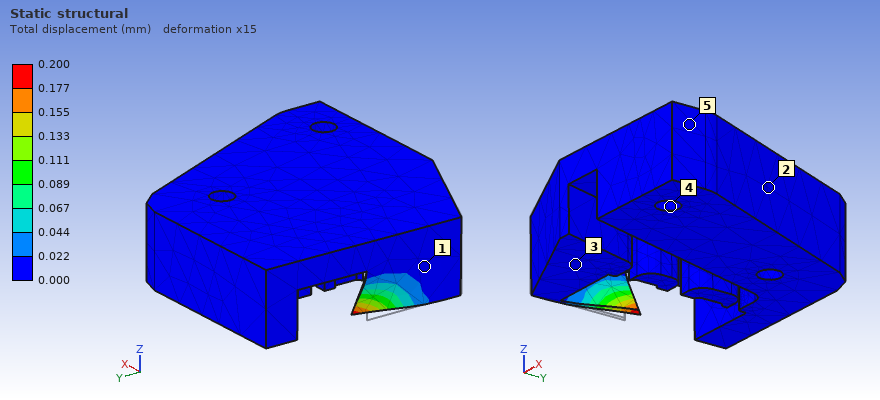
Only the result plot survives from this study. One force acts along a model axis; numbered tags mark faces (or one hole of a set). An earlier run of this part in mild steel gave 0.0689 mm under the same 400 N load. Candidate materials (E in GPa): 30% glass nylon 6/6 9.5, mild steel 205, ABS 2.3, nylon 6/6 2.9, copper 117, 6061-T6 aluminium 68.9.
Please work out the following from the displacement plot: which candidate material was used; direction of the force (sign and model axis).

6061-T6 aluminium
+X
